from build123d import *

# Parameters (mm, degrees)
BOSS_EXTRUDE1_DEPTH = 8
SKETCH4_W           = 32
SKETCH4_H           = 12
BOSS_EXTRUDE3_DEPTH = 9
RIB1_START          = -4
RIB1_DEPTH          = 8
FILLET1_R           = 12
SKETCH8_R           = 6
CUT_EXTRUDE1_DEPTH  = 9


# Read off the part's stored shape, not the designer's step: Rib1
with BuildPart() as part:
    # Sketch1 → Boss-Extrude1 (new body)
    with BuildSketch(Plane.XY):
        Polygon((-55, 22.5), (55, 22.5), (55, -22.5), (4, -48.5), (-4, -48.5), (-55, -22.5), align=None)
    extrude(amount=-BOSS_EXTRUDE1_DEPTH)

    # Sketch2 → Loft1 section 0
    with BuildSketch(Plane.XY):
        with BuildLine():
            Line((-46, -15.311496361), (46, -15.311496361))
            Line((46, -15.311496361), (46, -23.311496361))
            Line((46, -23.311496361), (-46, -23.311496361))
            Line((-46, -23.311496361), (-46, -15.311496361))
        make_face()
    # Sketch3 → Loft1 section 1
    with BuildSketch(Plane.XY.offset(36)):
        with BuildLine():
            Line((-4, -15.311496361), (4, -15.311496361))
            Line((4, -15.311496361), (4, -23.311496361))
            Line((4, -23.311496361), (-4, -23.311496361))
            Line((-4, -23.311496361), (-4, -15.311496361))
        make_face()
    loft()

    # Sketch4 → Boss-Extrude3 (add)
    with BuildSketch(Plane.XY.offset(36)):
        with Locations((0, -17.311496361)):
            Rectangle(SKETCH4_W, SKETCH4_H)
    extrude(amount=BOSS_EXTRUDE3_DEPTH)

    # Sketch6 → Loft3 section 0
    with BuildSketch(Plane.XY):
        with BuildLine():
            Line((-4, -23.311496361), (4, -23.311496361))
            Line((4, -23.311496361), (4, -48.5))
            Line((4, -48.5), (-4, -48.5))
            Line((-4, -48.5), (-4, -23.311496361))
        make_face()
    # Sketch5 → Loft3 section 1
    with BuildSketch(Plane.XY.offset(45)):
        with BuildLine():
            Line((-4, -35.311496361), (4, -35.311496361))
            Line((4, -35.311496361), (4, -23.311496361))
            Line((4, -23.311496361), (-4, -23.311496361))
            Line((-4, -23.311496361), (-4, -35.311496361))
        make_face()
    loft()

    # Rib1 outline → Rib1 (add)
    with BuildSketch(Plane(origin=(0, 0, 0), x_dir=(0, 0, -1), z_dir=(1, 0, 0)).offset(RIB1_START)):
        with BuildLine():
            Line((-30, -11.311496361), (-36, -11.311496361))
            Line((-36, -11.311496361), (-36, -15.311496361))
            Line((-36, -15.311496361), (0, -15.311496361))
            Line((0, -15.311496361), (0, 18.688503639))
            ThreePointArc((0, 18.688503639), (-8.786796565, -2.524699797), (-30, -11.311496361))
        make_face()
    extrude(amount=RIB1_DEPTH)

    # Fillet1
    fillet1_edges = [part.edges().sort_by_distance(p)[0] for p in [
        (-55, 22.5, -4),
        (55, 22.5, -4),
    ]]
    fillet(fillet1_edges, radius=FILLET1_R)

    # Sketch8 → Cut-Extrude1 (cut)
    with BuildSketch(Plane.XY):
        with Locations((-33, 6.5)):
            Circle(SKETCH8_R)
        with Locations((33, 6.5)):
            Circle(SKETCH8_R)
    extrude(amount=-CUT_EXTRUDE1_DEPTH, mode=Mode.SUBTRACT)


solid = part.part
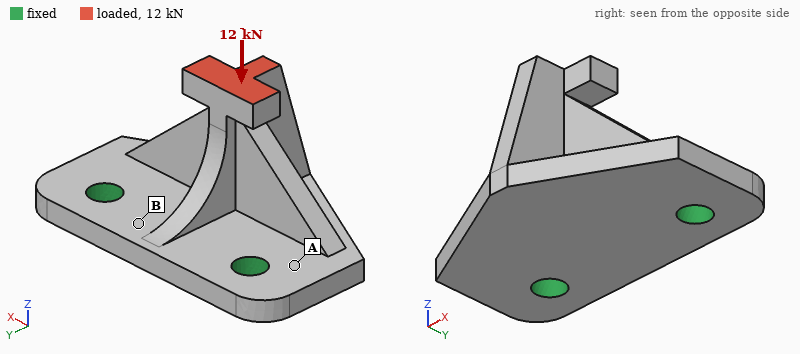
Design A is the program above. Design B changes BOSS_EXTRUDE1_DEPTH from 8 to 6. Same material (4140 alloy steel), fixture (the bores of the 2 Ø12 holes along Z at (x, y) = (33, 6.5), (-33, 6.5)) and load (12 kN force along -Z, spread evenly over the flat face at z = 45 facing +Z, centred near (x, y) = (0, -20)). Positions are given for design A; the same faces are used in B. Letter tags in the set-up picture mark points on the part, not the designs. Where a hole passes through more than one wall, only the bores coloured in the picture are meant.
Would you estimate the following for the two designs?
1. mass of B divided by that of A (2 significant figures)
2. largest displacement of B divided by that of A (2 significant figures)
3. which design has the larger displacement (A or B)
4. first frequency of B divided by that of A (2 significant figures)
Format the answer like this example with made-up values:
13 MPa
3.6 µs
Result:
0.84
2.0
B
0.75
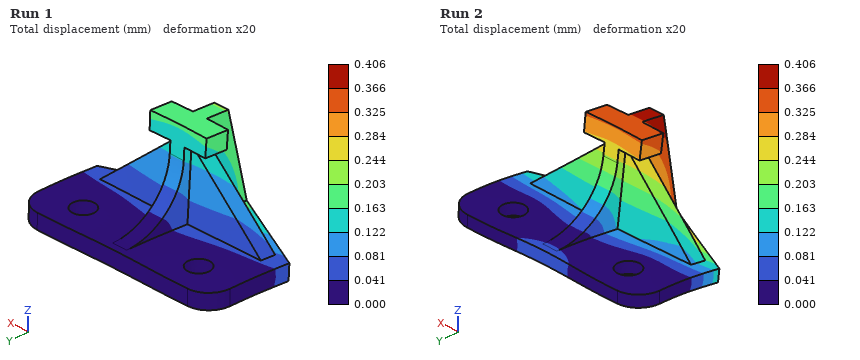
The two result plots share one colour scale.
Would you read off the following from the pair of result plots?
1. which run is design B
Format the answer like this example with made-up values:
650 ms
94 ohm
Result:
Run 2
